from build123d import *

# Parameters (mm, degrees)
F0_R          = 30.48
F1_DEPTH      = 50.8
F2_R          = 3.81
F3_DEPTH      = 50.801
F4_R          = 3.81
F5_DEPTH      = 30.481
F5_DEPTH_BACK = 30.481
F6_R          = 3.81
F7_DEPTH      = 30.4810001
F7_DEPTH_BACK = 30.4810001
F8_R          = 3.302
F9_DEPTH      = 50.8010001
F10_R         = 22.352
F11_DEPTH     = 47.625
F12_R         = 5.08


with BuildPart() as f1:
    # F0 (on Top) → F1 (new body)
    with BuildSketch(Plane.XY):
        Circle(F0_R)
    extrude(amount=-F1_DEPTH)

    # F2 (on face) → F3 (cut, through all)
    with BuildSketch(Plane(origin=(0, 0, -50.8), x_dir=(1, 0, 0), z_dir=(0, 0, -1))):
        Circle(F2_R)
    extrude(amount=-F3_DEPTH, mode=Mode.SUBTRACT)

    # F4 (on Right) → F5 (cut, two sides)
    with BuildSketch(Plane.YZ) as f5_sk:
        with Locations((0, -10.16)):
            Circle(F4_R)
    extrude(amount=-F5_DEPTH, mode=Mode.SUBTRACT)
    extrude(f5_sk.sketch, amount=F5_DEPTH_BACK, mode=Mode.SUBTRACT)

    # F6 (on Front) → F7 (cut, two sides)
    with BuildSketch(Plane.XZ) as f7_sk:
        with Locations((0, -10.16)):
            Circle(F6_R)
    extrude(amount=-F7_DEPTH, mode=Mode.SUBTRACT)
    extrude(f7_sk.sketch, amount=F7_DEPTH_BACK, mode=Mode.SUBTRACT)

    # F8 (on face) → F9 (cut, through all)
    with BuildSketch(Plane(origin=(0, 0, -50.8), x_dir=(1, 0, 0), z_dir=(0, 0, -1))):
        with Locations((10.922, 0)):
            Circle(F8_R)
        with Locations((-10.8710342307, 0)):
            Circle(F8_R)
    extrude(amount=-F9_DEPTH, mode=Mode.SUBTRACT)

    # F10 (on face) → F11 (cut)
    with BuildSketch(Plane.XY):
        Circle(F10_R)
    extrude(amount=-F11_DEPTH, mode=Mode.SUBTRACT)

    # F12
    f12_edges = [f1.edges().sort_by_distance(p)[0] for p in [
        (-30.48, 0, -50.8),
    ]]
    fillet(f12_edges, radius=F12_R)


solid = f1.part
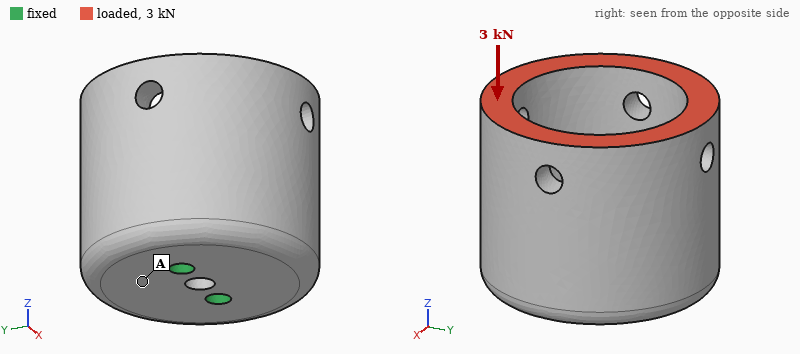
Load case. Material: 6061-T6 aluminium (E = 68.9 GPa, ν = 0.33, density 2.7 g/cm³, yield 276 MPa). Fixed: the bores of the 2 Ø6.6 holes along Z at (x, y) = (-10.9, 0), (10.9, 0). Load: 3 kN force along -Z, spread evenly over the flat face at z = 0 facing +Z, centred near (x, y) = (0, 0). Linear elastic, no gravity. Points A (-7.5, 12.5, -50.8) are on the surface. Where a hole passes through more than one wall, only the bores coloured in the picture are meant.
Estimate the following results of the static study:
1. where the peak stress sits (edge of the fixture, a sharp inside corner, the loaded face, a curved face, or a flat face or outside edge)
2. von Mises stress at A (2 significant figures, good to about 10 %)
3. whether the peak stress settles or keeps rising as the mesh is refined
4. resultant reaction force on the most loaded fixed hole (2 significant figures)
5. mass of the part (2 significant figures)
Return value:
edge of the fixture
15 MPa
keeps rising
1.5 kN
190 g
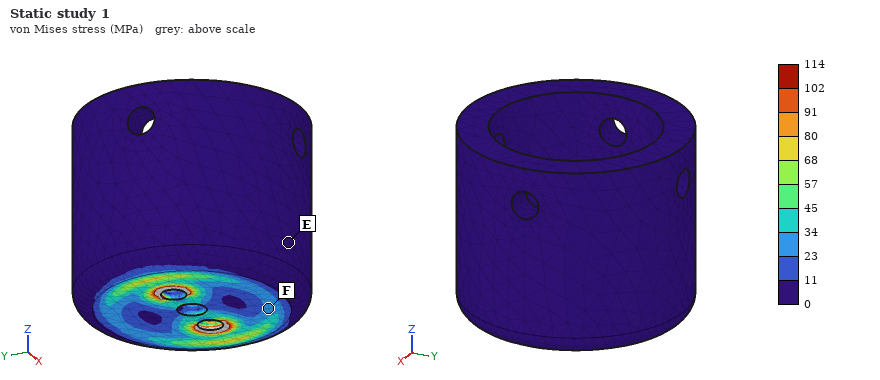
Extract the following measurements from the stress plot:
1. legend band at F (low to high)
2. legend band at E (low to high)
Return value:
23 to 34 MPa
0 to 11 MPa
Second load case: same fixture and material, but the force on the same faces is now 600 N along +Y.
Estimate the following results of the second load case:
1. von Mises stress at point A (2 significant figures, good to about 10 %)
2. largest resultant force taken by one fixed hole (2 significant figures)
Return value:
28 MPa
300 N
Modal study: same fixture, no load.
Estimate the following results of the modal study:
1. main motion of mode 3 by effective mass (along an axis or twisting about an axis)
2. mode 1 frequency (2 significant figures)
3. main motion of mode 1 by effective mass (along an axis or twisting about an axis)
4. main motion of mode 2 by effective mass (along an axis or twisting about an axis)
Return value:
along Z
740 Hz
along Y
along X
